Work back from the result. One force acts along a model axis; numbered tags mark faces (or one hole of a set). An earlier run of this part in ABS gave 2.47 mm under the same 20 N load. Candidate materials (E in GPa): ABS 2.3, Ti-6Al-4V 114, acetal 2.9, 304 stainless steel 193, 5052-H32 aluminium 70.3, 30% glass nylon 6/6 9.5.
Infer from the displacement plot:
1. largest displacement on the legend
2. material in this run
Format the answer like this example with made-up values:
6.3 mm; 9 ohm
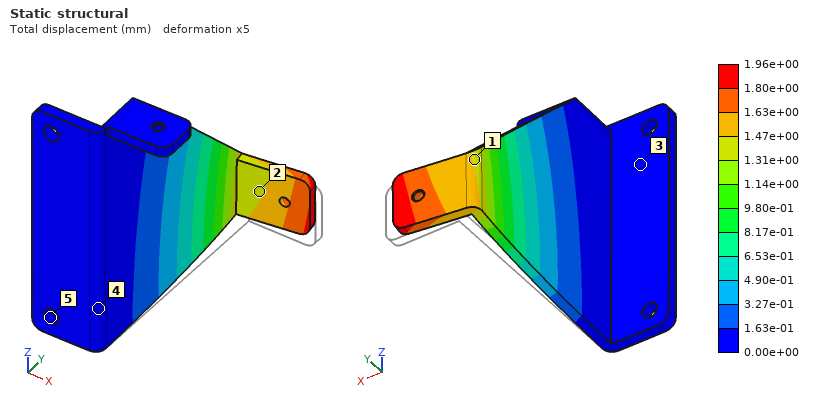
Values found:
1.96e+00 mm; acetal
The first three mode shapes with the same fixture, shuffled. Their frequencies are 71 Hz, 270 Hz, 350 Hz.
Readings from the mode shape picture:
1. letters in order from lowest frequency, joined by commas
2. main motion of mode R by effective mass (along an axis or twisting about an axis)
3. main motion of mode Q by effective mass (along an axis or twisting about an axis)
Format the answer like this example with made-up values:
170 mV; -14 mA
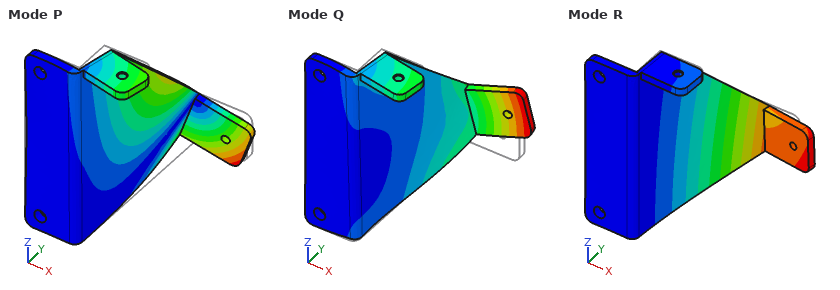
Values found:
R, P, Q; along X; along Z
